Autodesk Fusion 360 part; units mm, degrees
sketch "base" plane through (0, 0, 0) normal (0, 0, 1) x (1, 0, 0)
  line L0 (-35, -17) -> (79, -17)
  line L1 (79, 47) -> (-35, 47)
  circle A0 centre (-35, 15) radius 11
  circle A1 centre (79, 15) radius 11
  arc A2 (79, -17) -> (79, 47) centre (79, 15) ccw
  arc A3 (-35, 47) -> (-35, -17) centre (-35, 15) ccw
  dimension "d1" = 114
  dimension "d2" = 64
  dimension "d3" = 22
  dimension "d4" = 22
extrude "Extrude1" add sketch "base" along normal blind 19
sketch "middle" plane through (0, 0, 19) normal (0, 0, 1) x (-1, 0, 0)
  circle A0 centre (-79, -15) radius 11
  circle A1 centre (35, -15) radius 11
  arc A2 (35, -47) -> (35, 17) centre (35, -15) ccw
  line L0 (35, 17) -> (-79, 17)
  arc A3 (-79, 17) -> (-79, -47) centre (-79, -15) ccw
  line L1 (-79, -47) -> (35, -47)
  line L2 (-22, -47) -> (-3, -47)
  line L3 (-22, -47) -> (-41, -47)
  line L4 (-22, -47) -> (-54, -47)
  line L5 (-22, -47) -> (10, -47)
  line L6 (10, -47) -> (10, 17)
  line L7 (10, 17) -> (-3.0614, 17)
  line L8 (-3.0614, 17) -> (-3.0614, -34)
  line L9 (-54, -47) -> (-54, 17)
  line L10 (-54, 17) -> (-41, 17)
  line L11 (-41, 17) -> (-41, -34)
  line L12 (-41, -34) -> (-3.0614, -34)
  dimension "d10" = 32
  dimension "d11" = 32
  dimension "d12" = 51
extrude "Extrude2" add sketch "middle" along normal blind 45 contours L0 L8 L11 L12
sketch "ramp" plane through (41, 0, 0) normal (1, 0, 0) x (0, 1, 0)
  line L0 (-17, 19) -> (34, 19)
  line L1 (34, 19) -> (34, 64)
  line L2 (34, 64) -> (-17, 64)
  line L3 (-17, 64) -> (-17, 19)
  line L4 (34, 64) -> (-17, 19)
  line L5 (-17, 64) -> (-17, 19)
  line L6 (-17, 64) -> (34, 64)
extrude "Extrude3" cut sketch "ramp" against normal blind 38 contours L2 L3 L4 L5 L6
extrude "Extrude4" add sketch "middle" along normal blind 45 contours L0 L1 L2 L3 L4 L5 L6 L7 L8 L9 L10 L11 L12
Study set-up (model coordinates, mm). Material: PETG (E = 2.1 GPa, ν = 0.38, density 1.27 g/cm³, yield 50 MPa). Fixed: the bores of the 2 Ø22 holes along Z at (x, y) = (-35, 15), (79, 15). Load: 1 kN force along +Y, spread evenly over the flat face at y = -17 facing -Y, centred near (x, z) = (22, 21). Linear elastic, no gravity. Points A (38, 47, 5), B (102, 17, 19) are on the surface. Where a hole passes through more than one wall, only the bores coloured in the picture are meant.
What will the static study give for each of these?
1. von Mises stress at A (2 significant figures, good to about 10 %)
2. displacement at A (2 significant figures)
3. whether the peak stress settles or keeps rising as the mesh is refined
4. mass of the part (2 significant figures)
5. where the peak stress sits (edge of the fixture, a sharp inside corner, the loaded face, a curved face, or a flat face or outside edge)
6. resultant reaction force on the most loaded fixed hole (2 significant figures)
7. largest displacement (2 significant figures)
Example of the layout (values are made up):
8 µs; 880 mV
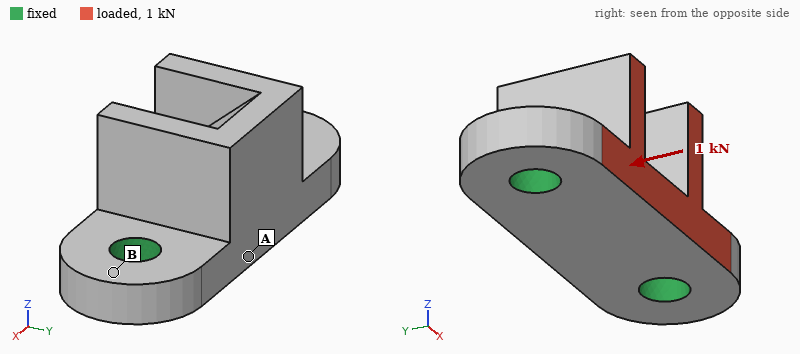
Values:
0.65 MPa; 38 µm; keeps rising; 410 g; edge of the fixture; 500 N; 99 µm
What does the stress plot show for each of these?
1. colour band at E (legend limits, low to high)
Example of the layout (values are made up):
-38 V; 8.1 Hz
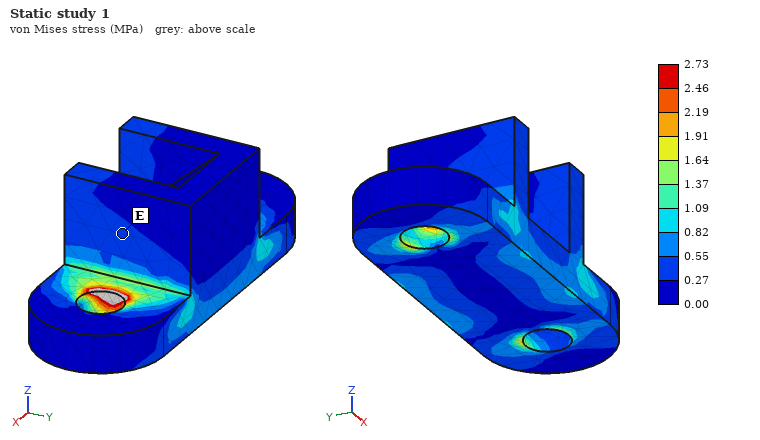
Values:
0.27 to 0.55 MPa
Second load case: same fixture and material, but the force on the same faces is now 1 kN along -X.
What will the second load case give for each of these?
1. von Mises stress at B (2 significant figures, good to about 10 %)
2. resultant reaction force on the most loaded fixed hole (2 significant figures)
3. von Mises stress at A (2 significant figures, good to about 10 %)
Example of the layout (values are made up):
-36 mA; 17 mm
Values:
0.13 MPa; 570 N; 0.17 MPa
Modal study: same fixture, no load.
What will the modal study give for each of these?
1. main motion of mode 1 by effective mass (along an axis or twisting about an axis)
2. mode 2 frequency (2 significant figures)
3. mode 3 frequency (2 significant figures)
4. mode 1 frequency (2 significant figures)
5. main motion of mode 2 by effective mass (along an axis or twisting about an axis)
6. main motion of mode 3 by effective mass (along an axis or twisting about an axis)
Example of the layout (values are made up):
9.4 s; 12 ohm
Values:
along Y; 1600 Hz; 1800 Hz; 880 Hz; along Z; along X
